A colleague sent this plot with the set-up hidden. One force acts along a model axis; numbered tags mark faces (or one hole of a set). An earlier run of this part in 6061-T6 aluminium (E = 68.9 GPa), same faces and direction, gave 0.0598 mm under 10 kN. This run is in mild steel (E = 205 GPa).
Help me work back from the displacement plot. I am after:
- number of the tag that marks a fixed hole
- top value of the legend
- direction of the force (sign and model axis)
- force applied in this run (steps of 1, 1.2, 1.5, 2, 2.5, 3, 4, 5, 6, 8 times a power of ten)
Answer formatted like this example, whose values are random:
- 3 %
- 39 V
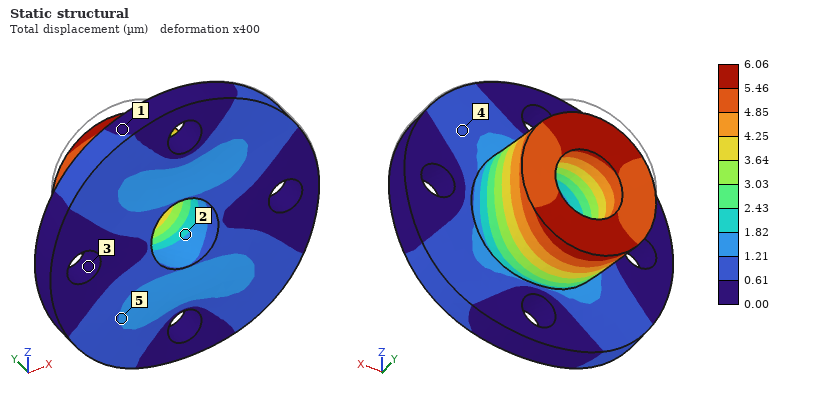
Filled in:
- 3
- 6.06 µm
- -Z
- 3 kN
